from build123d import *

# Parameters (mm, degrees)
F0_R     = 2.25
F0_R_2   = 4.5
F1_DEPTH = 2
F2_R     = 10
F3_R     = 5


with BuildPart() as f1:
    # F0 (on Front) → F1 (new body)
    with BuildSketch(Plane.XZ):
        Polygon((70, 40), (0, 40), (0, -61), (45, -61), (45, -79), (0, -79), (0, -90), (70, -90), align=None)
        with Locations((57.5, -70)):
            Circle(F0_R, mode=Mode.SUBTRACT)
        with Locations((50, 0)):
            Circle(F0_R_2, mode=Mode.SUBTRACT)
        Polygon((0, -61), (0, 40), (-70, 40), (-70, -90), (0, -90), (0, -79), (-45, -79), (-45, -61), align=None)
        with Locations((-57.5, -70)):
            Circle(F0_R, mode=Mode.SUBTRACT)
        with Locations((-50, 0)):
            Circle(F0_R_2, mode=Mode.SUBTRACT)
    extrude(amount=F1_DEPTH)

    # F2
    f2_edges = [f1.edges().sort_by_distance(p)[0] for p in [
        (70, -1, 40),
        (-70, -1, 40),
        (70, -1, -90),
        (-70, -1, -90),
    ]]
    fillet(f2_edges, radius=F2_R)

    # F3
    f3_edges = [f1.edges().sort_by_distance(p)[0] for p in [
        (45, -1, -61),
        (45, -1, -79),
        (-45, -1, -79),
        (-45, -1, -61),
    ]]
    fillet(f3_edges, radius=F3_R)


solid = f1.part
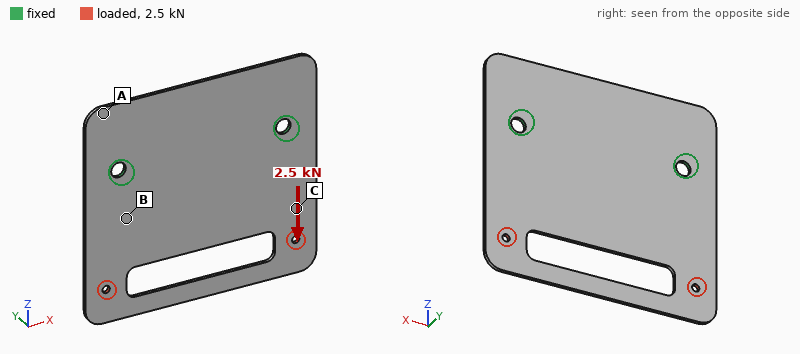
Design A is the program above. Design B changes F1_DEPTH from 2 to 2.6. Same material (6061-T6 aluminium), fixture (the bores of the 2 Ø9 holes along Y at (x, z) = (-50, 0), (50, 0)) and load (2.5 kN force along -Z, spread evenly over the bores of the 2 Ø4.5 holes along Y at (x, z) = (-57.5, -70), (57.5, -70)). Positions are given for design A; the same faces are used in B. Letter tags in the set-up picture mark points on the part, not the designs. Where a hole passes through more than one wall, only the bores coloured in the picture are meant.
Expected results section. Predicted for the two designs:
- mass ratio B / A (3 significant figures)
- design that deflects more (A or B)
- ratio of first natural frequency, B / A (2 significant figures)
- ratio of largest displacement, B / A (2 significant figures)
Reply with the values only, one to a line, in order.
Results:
1.30
A
1.3
0.77
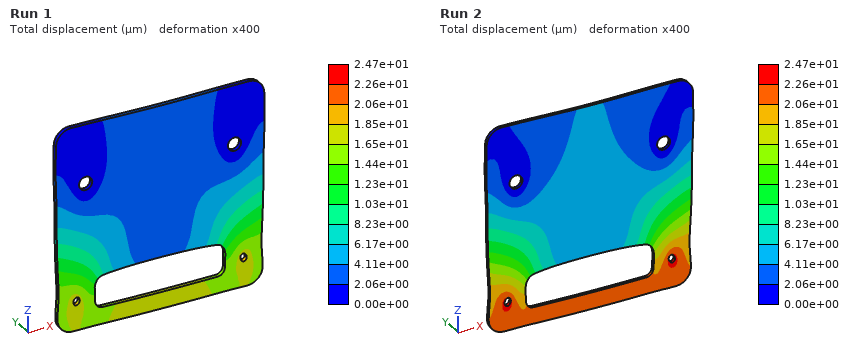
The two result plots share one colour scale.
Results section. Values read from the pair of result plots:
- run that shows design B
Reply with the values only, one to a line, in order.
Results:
Run 1
